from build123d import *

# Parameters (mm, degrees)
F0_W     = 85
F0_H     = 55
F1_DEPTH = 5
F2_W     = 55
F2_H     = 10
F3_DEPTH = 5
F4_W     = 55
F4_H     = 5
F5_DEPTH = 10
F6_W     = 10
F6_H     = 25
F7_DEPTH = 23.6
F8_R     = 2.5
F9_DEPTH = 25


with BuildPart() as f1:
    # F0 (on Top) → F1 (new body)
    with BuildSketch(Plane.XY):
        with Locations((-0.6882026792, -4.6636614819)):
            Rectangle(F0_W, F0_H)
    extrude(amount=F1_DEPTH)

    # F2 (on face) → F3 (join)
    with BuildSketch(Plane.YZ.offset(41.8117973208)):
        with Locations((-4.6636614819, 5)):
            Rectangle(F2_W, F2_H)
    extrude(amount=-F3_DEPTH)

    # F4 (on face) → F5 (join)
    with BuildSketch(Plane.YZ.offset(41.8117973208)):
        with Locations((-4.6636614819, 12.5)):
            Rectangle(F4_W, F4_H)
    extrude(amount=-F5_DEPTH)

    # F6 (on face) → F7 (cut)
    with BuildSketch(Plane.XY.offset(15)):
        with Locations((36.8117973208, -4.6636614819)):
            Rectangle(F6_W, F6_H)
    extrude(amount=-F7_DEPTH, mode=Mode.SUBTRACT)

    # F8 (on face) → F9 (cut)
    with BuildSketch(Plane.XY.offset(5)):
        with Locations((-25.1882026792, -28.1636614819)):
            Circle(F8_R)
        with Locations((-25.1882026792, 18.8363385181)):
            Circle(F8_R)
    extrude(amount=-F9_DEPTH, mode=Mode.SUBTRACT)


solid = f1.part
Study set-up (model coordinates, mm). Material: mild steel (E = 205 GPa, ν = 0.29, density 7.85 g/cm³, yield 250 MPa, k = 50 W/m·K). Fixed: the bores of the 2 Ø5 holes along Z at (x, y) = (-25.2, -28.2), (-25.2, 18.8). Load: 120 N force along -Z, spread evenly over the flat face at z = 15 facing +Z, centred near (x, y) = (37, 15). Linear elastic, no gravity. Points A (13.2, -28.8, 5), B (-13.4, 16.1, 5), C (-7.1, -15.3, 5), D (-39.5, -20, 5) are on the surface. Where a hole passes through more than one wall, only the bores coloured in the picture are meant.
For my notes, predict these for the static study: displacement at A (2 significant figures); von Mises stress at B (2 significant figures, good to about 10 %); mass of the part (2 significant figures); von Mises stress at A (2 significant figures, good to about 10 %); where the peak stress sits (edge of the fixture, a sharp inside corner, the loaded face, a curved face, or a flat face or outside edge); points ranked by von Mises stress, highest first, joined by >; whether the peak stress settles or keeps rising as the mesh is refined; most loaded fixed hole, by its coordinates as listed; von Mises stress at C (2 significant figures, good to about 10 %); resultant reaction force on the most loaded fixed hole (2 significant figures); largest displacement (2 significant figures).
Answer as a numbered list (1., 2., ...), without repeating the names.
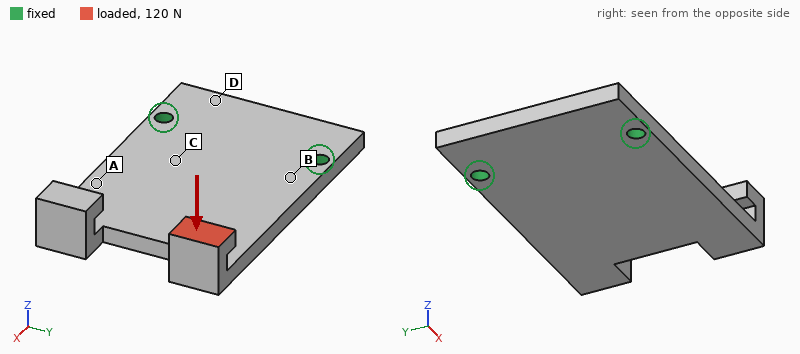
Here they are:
1. 0.034 mm
2. 33 MPa
3. 190 g
4. 11 MPa
5. edge of the fixture
6. B > C > A > D
7. keeps rising
8. (-25.2, 18.8)
9. 21 MPa
10. 110 N
11. 0.13 mm
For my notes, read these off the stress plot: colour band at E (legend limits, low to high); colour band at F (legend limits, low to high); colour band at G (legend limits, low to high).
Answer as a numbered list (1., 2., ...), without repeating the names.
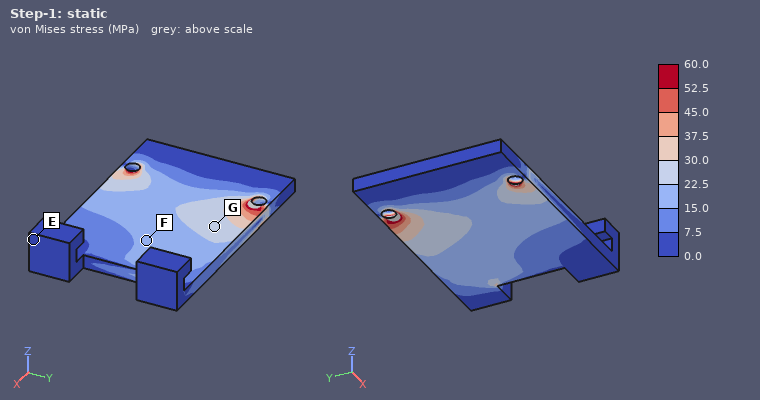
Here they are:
1. 0.0 to 7.5 MPa
2. 15.0 to 22.5 MPa
3. 22.5 to 30.0 MPa
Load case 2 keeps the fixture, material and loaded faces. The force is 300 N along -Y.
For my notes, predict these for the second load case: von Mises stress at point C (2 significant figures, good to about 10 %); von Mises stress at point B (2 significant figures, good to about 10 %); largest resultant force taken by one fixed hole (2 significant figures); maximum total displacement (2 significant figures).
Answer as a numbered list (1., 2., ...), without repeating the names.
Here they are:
1. 11 MPa
2. 15 MPa
3. 430 N
4. 52 µm
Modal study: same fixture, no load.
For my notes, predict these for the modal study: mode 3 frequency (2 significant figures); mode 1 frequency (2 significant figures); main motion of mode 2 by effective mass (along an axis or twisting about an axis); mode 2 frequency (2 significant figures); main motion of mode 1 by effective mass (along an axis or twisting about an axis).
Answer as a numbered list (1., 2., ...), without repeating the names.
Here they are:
1. 4400 Hz
2. 770 Hz
3. twisting about X
4. 1900 Hz
5. along Z
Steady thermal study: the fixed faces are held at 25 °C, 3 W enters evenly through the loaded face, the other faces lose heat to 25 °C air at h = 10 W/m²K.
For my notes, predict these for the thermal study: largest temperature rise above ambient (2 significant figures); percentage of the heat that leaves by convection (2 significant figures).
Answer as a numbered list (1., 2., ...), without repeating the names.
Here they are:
1. 31 K
2. 24 %
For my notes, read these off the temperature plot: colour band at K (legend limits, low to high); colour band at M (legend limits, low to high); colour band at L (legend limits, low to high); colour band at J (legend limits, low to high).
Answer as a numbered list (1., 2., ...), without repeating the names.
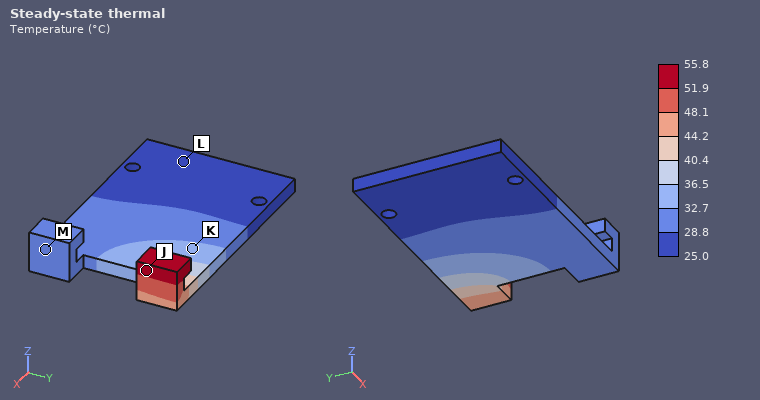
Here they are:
1. 32.7 to 36.5 °C
2. 28.8 to 32.7 °C
3. 25.0 to 28.8 °C
4. 51.9 to 55.8 °C
